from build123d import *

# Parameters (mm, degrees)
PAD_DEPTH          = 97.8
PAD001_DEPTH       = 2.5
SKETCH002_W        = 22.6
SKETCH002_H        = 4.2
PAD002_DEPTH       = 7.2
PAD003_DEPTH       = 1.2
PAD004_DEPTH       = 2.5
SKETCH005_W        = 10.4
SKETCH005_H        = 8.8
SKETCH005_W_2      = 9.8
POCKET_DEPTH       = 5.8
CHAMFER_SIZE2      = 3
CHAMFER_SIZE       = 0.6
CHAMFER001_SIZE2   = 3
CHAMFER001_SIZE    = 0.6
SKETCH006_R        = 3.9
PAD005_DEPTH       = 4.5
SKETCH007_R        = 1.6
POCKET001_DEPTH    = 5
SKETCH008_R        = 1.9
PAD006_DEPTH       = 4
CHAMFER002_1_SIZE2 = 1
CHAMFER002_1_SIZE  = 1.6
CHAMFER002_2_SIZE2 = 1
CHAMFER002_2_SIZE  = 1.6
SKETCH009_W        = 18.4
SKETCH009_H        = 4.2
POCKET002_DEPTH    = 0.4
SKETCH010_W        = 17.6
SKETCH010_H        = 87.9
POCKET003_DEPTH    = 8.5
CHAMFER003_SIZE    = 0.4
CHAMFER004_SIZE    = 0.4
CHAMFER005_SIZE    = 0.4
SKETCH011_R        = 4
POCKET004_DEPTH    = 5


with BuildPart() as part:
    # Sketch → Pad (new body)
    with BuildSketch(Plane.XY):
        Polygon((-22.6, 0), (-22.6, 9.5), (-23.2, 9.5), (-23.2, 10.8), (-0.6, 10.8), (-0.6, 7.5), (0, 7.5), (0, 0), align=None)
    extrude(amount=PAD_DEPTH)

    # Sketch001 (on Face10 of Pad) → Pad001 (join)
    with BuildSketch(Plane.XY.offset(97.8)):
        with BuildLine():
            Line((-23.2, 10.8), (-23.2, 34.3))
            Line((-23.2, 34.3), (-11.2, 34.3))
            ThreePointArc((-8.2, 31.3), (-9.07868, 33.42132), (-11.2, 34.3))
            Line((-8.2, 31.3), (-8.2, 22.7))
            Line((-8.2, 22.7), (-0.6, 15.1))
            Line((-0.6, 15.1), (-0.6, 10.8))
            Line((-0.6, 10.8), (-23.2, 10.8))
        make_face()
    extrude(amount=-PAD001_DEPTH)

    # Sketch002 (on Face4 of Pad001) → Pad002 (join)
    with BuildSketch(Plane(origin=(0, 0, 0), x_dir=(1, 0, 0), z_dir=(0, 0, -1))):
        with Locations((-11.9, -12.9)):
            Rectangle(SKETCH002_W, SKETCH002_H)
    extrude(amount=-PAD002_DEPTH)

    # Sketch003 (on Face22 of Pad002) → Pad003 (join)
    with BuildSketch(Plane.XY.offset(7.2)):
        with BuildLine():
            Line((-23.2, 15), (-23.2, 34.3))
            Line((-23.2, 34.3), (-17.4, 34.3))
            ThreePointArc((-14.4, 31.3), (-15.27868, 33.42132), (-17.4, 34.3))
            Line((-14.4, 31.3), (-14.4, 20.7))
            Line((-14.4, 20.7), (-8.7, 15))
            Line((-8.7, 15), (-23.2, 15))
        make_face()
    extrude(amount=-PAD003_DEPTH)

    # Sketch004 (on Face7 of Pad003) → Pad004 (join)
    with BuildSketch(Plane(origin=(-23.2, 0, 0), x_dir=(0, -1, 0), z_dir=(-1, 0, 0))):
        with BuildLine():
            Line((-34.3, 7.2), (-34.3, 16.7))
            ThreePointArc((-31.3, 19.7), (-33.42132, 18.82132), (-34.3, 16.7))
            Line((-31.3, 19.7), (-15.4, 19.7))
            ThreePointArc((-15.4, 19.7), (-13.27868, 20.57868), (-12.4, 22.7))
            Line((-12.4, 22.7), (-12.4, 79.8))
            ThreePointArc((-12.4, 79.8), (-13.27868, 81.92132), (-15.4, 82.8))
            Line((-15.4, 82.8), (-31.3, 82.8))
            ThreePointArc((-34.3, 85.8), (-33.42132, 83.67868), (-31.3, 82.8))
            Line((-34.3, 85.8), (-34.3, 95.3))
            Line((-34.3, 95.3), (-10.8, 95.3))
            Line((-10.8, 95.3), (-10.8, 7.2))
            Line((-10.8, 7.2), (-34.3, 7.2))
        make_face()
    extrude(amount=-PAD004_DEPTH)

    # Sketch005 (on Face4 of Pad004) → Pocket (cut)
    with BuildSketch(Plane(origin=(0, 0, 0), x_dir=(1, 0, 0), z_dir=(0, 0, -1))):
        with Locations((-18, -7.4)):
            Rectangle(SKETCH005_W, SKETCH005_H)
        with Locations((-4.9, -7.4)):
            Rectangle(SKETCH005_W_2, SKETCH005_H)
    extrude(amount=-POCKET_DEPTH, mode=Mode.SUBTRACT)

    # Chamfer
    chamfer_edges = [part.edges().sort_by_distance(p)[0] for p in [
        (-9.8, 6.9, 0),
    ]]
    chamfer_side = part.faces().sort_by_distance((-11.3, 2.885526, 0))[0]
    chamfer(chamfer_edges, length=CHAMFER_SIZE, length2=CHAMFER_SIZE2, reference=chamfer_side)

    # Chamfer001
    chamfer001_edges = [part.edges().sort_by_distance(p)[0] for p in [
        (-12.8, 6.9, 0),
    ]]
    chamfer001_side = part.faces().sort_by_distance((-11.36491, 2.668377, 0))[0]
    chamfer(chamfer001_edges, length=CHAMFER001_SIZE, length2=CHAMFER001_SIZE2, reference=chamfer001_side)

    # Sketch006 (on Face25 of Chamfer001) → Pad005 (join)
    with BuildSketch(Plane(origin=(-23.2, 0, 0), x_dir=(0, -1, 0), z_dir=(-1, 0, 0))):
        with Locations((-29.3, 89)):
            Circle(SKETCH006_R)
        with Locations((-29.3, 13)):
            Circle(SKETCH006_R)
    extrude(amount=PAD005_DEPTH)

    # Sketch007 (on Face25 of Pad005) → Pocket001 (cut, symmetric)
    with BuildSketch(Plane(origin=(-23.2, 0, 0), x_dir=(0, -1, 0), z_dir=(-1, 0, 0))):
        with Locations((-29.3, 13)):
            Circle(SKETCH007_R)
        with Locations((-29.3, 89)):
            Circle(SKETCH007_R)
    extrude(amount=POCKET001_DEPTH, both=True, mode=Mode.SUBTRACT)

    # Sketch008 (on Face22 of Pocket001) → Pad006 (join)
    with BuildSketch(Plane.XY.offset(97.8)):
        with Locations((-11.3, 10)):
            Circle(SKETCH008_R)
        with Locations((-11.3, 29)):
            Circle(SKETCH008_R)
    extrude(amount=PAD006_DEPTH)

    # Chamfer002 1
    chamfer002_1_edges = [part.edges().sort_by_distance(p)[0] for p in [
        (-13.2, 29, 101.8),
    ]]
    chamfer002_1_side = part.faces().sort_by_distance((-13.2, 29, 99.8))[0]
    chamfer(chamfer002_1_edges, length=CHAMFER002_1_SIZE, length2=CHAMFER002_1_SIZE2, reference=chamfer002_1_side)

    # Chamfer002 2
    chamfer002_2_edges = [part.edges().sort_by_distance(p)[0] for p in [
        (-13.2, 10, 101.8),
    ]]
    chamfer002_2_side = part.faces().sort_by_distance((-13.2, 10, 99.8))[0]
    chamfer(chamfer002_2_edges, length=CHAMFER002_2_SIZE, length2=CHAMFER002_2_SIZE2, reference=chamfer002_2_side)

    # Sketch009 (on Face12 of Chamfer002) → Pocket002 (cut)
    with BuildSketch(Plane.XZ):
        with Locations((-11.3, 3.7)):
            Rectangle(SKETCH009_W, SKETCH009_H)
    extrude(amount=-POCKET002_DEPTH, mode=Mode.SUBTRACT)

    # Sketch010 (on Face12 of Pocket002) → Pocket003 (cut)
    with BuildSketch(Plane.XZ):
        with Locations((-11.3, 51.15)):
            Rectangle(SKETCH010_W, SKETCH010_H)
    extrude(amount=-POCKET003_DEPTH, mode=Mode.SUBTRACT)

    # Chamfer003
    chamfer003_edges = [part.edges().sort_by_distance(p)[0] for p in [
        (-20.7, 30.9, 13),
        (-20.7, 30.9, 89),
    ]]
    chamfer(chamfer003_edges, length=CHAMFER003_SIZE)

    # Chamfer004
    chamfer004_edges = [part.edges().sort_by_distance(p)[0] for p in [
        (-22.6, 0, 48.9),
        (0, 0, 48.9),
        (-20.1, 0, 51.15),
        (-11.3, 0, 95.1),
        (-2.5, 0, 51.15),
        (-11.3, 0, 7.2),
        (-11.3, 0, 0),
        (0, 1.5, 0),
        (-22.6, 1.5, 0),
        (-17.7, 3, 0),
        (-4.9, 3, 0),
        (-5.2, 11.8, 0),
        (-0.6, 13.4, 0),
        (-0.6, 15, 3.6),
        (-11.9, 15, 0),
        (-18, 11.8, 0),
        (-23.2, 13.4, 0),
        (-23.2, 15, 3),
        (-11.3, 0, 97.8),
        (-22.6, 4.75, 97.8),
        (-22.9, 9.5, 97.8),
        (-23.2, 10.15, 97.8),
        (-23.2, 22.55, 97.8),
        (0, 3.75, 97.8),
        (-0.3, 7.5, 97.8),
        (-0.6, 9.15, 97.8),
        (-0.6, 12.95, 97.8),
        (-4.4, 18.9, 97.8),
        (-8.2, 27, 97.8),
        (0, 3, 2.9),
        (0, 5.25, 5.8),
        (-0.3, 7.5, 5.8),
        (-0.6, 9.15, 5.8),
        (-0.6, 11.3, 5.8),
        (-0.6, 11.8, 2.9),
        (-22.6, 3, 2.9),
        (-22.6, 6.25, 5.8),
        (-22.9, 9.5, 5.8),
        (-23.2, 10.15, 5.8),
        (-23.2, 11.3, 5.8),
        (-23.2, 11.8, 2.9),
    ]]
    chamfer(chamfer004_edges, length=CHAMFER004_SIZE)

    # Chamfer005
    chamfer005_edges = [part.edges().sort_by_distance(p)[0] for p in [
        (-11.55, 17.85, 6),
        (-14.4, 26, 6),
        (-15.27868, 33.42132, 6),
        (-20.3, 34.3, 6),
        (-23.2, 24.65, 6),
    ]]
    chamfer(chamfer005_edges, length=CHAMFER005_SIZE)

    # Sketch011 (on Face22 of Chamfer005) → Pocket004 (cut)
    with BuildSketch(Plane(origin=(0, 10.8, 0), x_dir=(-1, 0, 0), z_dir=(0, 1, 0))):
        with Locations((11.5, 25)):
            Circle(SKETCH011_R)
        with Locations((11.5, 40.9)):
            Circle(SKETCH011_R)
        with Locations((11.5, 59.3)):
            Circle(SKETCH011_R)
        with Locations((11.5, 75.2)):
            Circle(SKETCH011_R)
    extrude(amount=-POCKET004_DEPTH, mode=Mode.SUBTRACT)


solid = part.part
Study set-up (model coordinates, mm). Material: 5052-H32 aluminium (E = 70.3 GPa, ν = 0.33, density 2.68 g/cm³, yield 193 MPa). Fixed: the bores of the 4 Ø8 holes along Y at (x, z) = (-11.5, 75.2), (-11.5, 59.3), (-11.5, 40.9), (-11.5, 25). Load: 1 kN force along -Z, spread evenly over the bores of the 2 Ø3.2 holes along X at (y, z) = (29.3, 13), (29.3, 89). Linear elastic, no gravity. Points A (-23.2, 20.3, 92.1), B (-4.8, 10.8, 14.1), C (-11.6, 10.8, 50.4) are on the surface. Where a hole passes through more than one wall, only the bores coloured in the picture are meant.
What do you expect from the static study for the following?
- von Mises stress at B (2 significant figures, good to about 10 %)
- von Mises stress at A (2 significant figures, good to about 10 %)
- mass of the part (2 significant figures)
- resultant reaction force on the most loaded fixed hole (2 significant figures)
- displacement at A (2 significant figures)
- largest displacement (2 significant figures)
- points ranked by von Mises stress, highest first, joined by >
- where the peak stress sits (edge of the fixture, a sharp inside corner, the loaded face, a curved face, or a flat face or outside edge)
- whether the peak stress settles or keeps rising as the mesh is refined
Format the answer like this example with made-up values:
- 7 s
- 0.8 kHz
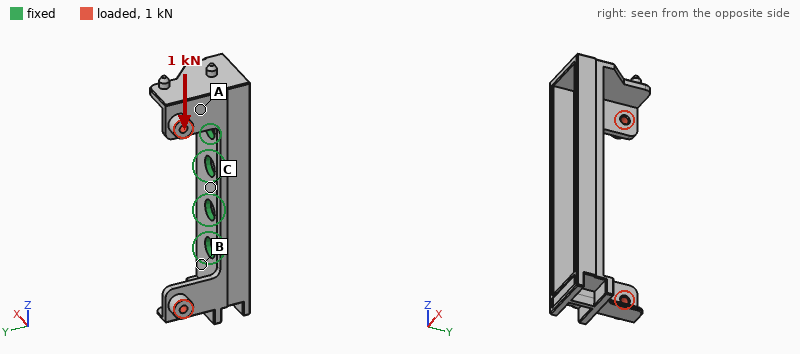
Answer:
- 30 MPa
- 68 MPa
- 35 g
- 820 N
- 0.15 mm
- 0.30 mm
- A > B > C
- a sharp inside corner
- keeps rising
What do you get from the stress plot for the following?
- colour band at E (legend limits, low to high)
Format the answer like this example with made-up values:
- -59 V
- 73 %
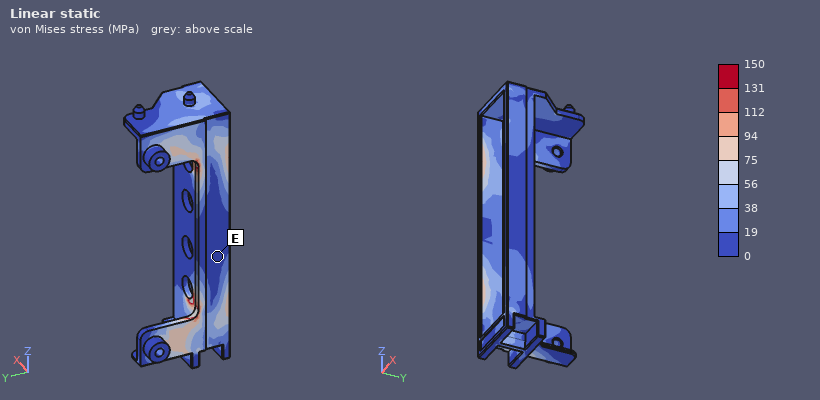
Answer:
- 0 to 19 MPa
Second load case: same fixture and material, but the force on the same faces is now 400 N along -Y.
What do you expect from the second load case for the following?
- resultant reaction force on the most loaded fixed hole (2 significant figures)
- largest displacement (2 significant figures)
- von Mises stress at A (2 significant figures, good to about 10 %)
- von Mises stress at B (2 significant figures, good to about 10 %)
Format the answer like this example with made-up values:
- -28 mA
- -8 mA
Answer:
- 280 N
- 0.11 mm
- 9.0 MPa
- 14 MPa
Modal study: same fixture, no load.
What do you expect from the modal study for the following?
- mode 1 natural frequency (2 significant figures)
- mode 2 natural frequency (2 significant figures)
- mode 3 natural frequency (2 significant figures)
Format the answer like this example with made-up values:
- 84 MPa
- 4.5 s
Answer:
- 2800 Hz
- 3300 Hz
- 4300 Hz
